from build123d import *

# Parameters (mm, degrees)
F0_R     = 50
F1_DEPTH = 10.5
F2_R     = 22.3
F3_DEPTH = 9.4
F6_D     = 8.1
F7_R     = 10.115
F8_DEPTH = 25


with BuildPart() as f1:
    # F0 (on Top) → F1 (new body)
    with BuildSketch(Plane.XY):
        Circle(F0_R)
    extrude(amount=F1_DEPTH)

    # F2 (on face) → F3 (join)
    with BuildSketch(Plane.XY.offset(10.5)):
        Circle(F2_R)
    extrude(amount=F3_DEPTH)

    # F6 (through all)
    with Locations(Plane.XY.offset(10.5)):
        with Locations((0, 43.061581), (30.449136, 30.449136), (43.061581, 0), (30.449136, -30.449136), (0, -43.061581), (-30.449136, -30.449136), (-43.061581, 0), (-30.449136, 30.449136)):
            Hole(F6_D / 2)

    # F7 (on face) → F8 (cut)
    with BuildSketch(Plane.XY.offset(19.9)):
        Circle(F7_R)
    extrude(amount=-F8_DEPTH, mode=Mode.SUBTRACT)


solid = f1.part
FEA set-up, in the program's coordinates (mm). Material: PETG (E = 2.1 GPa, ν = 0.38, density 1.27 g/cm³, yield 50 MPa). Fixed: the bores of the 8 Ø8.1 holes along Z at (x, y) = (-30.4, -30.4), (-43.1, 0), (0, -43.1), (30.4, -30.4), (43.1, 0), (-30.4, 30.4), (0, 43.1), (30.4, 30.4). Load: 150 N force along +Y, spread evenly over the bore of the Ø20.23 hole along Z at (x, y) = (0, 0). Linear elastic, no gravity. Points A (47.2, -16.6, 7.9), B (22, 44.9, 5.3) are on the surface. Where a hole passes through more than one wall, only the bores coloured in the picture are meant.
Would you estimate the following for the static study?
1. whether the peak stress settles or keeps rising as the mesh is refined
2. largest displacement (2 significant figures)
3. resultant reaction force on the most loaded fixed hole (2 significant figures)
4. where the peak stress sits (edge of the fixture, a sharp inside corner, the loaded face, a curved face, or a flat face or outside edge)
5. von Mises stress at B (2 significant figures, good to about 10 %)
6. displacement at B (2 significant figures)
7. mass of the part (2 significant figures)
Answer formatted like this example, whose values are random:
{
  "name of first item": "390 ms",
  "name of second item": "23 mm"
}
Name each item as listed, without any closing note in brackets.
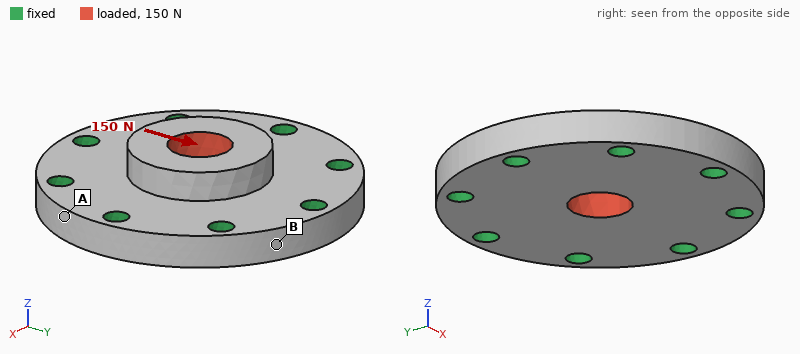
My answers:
{
  "whether the peak stress settles or keeps rising as the mesh is refined": "keeps rising",
  "largest displacement": "3.6 µm",
  "resultant reaction force on the most loaded fixed hole": "32 N",
  "where the peak stress sits": "edge of the fixture",
  "von Mises stress at B": "0.065 MPa",
  "displacement at B": "0.58 µm",
  "mass of the part": "110 g"
}
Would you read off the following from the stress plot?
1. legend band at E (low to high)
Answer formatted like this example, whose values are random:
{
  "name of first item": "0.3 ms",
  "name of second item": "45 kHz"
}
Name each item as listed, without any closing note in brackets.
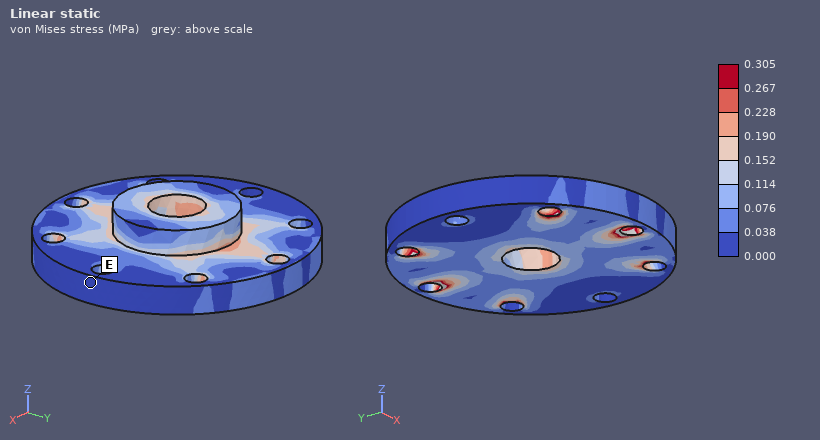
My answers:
{
  "legend band at E": "0.000 to 0.038 MPa"
}
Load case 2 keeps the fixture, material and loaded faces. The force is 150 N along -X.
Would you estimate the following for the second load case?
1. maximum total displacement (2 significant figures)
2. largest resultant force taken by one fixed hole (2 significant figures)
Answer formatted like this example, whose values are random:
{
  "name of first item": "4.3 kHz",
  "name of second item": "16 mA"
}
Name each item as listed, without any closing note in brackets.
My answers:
{
  "maximum total displacement": "3.6 µm",
  "largest resultant force taken by one fixed hole": "32 N"
}
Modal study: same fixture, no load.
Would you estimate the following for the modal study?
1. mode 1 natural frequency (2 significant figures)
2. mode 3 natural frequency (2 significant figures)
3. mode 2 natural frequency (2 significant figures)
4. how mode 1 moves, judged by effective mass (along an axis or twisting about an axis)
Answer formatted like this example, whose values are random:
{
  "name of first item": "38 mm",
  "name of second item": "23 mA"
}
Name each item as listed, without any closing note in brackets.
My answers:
{
  "mode 1 natural frequency": "3200 Hz",
  "mode 3 natural frequency": "5100 Hz",
  "mode 2 natural frequency": "5100 Hz",
  "how mode 1 moves, judged by effective mass": "along Z"
}
